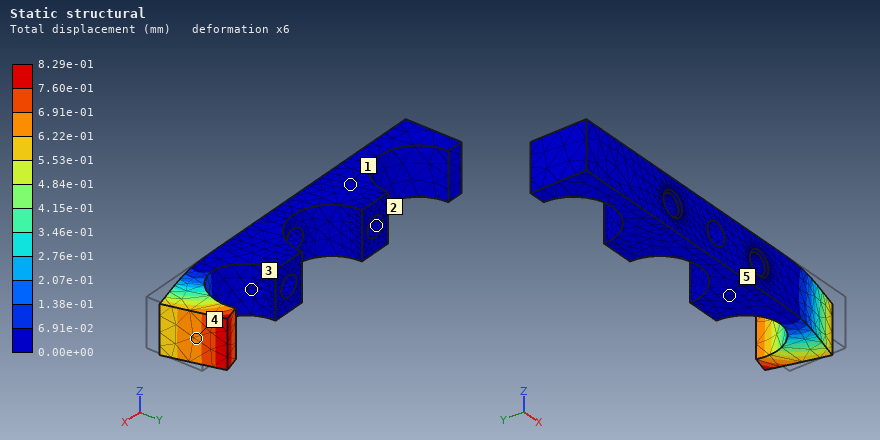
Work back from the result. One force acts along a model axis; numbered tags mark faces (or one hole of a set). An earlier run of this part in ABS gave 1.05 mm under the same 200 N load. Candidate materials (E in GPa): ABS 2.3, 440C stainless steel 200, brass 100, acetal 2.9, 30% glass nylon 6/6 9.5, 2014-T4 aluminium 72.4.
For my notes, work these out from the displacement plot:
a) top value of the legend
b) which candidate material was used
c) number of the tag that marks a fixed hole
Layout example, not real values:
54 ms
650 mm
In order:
8.29e-01 mm
acetal
2
